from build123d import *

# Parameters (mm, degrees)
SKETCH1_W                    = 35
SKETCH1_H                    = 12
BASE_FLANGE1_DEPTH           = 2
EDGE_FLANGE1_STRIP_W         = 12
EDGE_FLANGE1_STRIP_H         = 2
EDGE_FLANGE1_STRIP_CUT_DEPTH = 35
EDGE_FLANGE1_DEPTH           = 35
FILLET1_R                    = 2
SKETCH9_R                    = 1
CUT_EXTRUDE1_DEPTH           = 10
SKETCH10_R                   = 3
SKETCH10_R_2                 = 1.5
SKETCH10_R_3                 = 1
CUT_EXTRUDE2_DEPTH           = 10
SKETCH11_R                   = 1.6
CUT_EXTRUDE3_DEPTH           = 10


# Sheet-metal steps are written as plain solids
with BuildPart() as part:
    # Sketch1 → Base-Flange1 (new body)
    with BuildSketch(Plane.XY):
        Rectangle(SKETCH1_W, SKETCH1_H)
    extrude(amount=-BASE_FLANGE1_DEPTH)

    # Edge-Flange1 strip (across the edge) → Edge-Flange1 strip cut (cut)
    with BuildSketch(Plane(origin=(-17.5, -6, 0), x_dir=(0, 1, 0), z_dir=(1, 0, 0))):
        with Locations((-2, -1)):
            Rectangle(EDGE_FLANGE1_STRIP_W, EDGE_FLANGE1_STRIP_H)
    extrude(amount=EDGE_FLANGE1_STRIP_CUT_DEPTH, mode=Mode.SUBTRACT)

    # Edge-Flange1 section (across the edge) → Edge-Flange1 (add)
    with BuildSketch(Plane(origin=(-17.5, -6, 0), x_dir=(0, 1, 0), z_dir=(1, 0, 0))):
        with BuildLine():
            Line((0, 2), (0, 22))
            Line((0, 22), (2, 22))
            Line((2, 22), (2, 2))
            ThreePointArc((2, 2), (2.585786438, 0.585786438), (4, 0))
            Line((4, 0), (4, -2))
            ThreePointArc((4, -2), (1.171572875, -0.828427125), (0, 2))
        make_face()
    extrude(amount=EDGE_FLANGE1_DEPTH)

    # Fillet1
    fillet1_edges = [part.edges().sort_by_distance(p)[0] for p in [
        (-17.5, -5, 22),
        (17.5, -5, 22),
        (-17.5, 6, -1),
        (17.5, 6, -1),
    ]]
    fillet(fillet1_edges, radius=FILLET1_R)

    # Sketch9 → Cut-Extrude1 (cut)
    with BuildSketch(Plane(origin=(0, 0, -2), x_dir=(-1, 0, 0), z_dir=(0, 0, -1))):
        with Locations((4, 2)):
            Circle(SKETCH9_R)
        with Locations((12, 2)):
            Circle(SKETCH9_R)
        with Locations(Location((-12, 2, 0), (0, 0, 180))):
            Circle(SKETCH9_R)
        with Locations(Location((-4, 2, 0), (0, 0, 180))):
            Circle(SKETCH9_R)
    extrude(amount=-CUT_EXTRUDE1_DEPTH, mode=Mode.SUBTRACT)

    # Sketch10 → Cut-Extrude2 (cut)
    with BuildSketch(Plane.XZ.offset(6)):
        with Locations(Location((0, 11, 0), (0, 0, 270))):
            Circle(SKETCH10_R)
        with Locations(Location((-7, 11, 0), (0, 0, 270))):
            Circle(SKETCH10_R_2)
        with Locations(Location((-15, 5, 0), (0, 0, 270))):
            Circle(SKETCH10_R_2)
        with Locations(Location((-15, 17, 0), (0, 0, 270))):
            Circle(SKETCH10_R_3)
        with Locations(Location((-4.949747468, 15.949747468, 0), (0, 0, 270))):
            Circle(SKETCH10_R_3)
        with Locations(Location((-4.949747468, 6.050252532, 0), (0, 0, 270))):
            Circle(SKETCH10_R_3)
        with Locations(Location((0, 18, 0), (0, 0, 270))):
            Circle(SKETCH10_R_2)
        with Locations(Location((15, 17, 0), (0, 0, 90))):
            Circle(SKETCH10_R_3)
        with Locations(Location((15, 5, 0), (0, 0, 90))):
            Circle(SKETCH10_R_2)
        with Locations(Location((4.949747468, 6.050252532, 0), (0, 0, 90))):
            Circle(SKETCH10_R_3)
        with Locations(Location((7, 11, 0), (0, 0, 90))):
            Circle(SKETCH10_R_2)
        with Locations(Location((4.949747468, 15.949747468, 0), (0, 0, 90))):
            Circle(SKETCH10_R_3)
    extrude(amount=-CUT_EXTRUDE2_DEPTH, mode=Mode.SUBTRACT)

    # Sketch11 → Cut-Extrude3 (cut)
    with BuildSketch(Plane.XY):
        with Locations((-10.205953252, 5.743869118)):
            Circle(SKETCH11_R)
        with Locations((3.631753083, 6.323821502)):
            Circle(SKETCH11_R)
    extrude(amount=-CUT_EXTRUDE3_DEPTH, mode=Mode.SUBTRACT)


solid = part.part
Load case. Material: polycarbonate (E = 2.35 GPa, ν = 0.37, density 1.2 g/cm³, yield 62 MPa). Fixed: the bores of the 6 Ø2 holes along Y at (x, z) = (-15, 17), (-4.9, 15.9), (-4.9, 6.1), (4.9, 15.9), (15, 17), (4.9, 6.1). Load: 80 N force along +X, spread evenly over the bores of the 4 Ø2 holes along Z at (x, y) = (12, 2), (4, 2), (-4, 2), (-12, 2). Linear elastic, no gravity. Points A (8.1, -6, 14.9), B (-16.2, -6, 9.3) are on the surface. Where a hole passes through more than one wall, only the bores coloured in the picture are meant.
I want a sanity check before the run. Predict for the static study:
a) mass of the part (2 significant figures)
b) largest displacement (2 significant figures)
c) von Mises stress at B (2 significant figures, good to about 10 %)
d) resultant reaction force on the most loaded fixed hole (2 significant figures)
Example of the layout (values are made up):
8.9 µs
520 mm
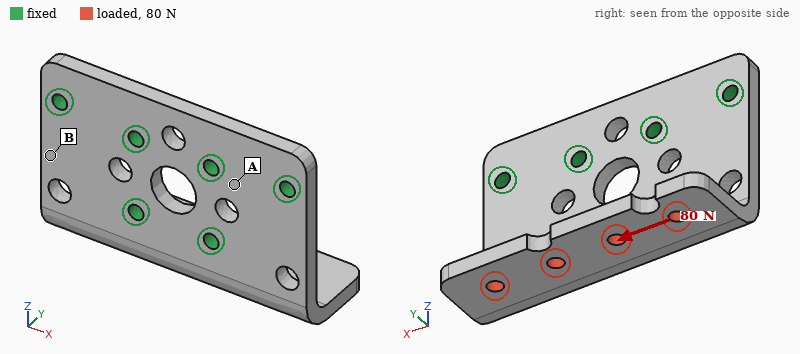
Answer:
2.5 g
0.47 mm
6.1 MPa
58 N
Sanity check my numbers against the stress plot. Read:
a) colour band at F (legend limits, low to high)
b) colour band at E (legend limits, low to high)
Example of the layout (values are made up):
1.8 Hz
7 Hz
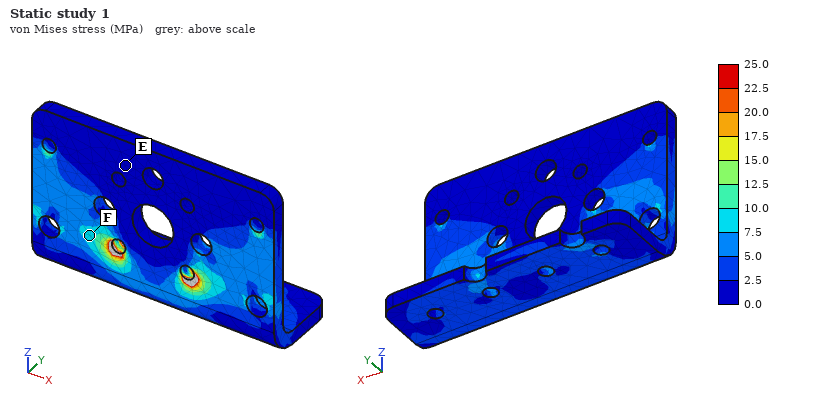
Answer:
7.5 to 10.0 MPa
0.0 to 2.5 MPa
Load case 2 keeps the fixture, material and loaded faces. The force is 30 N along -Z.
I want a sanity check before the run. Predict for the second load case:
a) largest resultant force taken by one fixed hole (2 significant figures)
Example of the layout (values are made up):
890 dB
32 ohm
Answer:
11 N
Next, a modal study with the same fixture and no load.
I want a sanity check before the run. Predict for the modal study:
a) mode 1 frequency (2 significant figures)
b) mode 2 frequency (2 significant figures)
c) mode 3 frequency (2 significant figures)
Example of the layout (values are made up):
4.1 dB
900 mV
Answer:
1900 Hz
2000 Hz
3900 Hz
